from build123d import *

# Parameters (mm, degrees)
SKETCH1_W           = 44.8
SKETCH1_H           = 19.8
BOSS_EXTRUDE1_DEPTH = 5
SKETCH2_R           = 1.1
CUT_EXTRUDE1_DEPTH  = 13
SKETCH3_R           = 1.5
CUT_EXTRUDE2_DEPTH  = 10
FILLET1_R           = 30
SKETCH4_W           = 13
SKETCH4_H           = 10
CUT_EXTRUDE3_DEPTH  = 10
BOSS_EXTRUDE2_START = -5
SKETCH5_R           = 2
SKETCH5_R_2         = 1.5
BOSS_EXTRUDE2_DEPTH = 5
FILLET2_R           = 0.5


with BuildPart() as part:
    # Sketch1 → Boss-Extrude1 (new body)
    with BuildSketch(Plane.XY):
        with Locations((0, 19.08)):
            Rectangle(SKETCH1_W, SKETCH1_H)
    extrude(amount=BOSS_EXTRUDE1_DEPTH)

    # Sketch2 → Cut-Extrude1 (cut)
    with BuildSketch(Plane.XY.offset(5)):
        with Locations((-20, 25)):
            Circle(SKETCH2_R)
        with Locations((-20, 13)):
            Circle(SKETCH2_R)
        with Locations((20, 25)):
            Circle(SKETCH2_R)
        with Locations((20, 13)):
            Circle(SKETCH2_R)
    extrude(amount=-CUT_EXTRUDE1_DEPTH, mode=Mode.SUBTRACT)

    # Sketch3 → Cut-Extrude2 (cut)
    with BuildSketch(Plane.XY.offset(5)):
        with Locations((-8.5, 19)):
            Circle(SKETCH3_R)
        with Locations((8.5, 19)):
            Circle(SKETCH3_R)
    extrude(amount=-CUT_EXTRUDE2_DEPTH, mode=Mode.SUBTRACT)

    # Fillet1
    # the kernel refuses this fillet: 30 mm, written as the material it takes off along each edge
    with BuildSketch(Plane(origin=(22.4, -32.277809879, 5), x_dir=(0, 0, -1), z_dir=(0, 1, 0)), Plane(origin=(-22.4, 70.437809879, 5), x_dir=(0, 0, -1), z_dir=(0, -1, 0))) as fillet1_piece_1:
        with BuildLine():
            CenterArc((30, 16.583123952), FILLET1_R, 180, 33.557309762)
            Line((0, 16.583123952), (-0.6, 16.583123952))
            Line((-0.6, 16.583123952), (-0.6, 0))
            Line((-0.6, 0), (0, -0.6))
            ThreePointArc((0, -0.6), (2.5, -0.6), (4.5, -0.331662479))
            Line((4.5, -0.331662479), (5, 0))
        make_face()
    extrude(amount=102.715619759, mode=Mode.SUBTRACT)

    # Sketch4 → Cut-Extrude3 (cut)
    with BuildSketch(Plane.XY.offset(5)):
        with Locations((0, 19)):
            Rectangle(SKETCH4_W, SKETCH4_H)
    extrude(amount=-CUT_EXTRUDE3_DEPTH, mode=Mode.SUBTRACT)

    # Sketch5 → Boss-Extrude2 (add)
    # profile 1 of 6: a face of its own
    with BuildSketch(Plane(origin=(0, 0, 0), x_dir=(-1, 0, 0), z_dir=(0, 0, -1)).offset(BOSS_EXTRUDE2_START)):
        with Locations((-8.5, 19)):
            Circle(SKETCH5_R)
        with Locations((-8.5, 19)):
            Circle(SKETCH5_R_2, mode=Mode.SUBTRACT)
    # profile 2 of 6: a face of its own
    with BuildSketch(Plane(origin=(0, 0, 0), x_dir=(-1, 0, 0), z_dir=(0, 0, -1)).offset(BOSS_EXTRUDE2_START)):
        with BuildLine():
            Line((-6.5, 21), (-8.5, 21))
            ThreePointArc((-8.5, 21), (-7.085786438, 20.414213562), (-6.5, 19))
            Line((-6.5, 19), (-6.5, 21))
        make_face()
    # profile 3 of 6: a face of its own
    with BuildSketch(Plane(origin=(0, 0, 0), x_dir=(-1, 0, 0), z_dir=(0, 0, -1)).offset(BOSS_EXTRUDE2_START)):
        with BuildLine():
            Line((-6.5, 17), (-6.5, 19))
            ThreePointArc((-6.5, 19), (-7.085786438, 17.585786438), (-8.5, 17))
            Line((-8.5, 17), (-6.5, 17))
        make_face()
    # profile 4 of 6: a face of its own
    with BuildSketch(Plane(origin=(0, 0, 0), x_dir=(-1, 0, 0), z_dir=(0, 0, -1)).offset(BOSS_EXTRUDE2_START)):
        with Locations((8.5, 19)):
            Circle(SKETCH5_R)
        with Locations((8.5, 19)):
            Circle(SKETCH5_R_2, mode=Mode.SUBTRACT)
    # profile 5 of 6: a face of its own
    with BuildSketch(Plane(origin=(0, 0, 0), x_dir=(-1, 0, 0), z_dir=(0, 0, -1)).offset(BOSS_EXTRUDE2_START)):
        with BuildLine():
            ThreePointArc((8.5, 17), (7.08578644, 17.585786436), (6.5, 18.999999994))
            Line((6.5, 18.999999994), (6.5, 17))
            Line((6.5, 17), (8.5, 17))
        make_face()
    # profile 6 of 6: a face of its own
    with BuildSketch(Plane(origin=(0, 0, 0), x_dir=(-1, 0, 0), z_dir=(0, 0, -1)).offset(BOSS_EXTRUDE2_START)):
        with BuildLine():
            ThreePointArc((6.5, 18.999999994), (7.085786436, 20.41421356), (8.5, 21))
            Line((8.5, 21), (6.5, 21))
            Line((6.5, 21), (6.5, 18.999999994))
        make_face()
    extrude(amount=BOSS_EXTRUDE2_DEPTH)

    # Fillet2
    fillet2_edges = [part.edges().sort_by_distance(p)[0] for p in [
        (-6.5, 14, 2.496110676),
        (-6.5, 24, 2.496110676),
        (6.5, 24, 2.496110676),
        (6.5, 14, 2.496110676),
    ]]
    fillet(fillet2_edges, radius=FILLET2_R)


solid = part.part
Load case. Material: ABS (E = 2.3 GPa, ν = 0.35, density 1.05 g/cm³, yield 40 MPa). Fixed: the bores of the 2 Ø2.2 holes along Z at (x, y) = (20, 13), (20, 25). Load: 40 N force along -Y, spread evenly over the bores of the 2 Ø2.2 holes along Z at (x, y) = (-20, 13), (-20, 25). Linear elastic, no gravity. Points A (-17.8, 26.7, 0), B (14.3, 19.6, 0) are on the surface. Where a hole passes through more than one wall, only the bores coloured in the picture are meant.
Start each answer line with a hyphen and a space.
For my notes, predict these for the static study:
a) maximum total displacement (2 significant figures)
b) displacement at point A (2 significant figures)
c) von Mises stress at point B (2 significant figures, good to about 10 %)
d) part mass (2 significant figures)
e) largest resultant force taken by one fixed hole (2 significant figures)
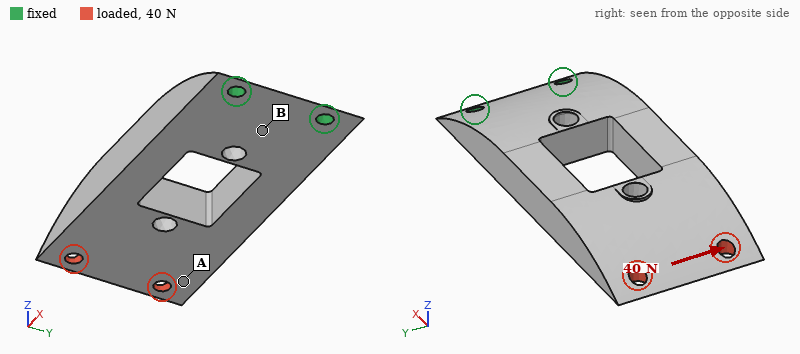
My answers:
- 0.48 mm
- 0.42 mm
- 8.3 MPa
- 2.8 g
- 120 N
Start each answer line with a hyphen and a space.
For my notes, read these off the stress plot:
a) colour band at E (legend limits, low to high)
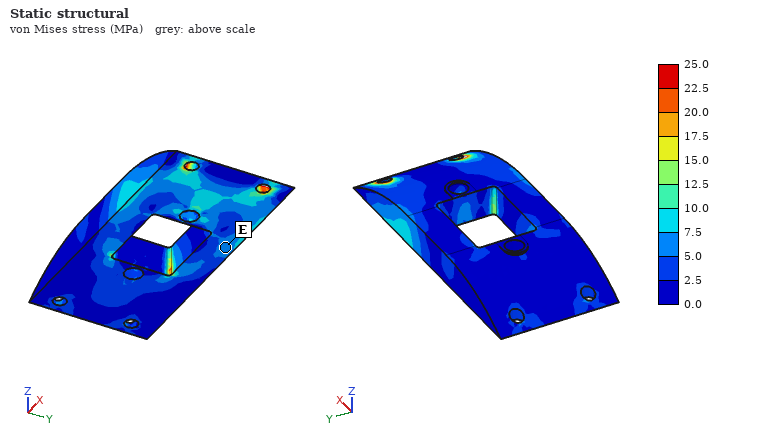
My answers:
- 5.0 to 7.5 MPa
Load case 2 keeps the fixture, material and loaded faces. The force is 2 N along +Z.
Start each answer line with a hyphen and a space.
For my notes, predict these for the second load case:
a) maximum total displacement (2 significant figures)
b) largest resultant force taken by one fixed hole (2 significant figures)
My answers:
- 0.49 mm
- 1.0 N
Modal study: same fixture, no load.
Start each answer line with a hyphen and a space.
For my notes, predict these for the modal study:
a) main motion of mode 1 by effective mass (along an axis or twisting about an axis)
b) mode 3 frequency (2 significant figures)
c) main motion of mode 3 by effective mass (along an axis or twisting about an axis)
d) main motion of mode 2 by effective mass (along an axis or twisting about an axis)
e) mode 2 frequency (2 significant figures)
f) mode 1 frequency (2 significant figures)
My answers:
- along Z
- 2000 Hz
- along Y
- along Y
- 1600 Hz
- 370 Hz
